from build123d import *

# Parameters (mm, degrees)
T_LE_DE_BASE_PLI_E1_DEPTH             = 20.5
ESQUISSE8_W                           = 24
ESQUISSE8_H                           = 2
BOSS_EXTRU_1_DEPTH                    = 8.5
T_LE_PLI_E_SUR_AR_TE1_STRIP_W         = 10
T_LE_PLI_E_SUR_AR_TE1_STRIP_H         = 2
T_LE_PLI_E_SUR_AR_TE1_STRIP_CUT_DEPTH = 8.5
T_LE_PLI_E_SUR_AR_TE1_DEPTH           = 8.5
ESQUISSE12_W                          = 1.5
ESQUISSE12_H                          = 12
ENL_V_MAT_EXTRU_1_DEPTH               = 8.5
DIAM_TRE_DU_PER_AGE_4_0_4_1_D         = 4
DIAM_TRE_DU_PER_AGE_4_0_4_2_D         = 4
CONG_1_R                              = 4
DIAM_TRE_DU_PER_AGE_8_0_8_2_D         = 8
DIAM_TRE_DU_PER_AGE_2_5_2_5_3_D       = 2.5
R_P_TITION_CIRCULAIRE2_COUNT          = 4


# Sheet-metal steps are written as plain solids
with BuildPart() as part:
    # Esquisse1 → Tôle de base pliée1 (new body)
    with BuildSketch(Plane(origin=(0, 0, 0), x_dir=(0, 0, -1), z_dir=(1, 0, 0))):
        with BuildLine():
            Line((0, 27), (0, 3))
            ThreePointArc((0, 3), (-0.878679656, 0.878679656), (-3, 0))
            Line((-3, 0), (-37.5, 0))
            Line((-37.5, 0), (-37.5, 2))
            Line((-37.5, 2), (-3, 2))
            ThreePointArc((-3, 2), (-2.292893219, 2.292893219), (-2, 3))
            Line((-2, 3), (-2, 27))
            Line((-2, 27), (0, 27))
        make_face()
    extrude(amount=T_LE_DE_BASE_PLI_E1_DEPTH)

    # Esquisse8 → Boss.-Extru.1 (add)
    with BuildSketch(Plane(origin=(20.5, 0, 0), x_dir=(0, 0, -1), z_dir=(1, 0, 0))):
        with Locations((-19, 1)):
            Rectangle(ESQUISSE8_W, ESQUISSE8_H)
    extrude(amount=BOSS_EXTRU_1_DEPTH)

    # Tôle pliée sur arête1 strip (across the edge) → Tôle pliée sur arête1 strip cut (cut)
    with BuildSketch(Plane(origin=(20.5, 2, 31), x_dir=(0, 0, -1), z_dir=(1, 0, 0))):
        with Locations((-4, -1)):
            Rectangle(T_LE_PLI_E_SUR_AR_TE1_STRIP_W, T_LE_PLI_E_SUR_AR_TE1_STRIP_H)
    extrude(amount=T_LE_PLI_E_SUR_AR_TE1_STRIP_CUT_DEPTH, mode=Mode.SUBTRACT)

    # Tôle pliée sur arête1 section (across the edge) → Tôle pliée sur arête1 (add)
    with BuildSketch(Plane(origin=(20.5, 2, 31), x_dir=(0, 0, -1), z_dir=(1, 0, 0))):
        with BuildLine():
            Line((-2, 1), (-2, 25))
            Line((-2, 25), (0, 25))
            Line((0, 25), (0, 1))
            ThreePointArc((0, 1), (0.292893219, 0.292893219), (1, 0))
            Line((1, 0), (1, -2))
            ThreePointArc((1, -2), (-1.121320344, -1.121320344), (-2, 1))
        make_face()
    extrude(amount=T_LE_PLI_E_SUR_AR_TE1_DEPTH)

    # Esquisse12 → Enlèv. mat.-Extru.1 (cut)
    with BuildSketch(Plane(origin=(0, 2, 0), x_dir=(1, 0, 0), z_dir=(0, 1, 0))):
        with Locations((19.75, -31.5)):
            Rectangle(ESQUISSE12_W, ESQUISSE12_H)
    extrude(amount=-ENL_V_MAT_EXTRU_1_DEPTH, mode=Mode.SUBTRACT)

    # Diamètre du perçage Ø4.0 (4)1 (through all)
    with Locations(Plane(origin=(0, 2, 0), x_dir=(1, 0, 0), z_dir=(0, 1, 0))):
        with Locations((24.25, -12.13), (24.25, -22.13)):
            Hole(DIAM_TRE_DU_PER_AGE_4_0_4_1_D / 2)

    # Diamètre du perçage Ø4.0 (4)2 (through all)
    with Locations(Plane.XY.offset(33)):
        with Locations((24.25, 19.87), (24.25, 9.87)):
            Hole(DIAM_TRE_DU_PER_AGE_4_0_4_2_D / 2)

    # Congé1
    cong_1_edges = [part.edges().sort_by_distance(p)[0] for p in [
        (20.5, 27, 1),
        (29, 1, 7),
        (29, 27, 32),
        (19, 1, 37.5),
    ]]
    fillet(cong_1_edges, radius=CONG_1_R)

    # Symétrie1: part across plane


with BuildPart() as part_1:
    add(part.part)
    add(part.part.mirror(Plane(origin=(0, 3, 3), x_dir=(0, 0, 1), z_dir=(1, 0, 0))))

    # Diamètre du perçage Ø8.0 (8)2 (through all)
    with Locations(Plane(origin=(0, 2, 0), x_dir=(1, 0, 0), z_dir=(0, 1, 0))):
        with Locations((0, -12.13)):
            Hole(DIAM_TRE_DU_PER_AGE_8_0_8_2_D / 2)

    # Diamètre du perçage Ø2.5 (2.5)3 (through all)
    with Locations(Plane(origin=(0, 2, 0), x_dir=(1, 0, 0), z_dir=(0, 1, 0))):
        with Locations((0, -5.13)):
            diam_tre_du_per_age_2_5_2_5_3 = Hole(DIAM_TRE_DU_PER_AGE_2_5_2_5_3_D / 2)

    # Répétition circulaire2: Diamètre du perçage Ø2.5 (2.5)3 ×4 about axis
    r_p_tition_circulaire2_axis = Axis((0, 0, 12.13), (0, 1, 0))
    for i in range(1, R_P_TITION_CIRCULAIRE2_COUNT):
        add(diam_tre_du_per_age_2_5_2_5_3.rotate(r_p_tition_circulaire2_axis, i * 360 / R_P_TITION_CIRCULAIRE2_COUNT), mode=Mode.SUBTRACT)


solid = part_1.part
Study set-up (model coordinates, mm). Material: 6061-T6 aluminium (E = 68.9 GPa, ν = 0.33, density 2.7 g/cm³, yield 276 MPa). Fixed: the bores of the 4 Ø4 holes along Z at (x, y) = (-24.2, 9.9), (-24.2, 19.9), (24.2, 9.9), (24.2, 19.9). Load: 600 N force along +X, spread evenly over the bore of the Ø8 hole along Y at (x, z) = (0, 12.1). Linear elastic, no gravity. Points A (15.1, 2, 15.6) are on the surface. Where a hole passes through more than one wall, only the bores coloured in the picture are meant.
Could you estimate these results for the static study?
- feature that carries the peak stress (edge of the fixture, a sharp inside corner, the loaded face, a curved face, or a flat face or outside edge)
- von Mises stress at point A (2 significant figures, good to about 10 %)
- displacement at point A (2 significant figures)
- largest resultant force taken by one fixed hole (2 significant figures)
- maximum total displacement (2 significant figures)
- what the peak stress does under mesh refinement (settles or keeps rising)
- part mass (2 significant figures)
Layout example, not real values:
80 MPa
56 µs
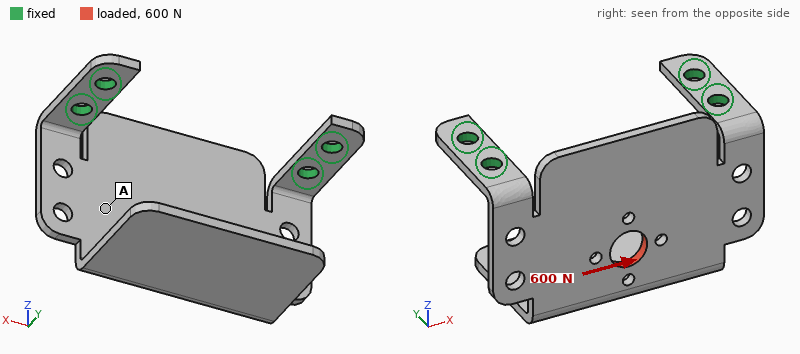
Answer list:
edge of the fixture
28 MPa
0.11 mm
420 N
0.27 mm
keeps rising
17 g
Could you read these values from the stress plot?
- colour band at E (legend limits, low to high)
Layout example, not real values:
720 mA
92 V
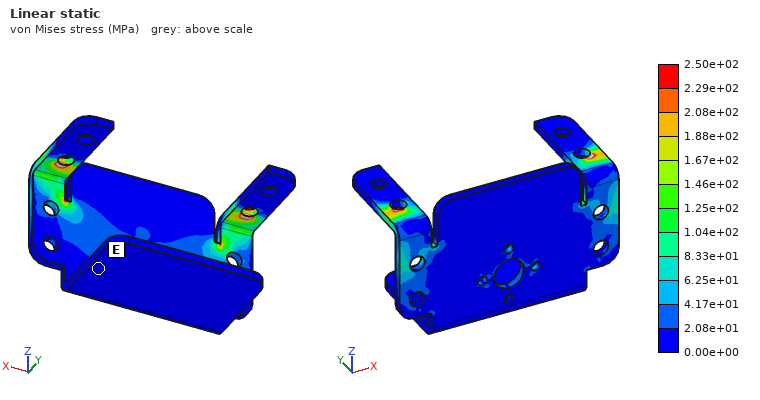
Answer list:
0.00e+00 to 2.08e+01 MPa
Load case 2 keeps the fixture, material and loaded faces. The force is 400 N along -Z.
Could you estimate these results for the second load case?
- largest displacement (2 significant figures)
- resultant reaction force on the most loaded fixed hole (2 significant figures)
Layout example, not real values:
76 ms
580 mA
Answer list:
0.53 mm
210 N
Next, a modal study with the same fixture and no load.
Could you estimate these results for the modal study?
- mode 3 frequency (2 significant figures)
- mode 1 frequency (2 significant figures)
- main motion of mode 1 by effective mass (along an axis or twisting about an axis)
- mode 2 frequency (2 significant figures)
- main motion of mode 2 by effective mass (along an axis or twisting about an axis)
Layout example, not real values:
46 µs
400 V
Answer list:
1400 Hz
370 Hz
along Y
1100 Hz
along X
